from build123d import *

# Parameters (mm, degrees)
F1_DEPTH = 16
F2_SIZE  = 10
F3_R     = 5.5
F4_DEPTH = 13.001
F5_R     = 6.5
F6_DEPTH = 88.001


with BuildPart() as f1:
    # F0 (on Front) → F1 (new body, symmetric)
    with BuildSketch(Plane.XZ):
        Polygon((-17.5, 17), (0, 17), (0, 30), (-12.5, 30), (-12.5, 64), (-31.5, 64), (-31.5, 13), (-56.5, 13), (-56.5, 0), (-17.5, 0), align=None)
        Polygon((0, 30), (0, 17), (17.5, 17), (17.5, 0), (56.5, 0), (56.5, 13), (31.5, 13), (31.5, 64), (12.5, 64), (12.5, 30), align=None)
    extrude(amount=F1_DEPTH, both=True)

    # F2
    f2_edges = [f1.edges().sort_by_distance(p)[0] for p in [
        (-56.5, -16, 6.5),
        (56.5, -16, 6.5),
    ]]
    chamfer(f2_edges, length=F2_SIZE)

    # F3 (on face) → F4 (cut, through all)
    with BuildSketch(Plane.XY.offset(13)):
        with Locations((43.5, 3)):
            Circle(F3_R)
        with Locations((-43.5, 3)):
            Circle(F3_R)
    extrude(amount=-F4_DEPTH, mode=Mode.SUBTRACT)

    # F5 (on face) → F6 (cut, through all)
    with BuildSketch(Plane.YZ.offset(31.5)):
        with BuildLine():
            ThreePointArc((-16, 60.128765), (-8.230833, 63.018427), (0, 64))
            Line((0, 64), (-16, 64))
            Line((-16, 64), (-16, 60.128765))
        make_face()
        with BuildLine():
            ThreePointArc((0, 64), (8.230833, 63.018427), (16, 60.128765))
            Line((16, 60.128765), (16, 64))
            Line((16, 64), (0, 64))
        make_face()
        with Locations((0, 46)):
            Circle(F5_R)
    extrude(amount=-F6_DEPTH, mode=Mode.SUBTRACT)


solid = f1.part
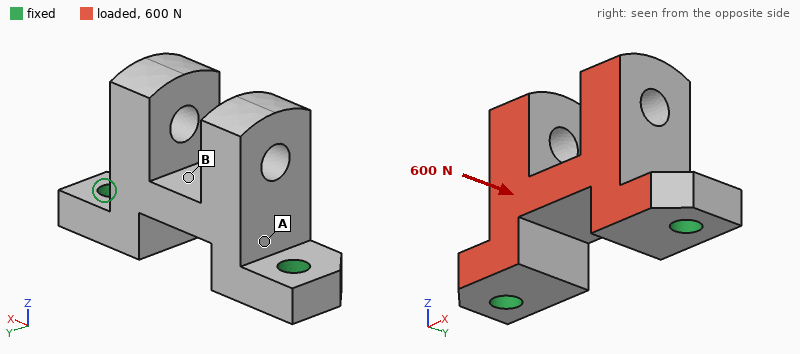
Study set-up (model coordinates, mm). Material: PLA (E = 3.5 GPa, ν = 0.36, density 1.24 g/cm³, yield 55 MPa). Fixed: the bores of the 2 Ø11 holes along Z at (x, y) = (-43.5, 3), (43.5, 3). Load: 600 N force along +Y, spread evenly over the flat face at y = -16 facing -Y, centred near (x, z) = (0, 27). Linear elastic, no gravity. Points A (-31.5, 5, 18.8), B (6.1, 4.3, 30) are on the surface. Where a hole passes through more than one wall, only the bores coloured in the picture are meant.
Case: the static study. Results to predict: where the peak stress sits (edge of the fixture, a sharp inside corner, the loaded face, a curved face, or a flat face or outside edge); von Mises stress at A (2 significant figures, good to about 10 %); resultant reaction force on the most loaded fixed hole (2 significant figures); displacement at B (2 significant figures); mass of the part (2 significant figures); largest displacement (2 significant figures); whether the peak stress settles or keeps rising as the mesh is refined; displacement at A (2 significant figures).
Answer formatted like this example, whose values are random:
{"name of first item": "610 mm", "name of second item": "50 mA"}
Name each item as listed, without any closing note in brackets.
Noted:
{"where the peak stress sits": "edge of the fixture", "von Mises stress at A": "2.4 MPa", "resultant reaction force on the most loaded fixed hole": "300 N", "displacement at B": "0.11 mm", "mass of the part": "120 g", "largest displacement": "0.24 mm", "whether the peak stress settles or keeps rising as the mesh is refined": "keeps rising", "displacement at A": "0.057 mm"}
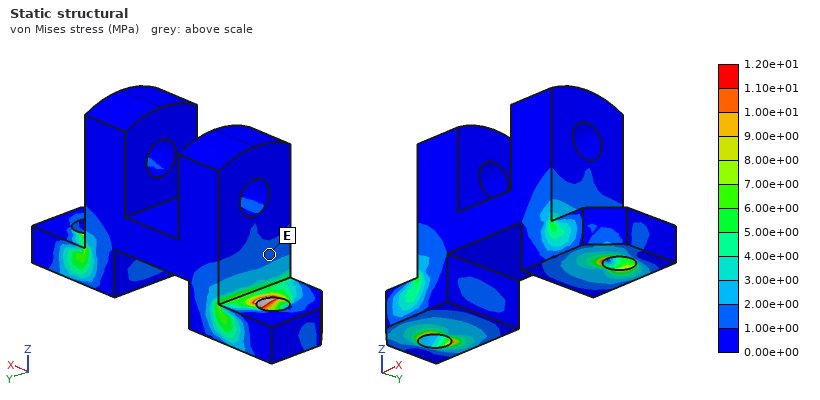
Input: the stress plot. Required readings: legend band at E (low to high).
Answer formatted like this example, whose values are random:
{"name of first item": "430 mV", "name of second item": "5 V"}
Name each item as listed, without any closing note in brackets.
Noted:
{"legend band at E": "1.00e+00 to 2.00e+00 MPa"}
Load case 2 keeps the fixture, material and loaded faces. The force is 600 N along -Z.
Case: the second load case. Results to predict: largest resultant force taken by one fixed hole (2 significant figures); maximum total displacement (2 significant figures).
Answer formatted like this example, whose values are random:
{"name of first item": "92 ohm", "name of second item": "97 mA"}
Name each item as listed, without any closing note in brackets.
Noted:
{"largest resultant force taken by one fixed hole": "340 N", "maximum total displacement": "0.18 mm"}
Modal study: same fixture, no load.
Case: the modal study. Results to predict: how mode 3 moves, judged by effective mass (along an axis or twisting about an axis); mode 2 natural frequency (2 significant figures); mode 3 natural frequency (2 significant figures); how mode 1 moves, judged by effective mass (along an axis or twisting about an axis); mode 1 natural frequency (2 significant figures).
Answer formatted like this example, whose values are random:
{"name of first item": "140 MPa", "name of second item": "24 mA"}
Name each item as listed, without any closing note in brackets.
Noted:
{"how mode 3 moves, judged by effective mass": "along X", "mode 2 natural frequency": "1500 Hz", "mode 3 natural frequency": "1900 Hz", "how mode 1 moves, judged by effective mass": "along Y", "mode 1 natural frequency": "920 Hz"}
